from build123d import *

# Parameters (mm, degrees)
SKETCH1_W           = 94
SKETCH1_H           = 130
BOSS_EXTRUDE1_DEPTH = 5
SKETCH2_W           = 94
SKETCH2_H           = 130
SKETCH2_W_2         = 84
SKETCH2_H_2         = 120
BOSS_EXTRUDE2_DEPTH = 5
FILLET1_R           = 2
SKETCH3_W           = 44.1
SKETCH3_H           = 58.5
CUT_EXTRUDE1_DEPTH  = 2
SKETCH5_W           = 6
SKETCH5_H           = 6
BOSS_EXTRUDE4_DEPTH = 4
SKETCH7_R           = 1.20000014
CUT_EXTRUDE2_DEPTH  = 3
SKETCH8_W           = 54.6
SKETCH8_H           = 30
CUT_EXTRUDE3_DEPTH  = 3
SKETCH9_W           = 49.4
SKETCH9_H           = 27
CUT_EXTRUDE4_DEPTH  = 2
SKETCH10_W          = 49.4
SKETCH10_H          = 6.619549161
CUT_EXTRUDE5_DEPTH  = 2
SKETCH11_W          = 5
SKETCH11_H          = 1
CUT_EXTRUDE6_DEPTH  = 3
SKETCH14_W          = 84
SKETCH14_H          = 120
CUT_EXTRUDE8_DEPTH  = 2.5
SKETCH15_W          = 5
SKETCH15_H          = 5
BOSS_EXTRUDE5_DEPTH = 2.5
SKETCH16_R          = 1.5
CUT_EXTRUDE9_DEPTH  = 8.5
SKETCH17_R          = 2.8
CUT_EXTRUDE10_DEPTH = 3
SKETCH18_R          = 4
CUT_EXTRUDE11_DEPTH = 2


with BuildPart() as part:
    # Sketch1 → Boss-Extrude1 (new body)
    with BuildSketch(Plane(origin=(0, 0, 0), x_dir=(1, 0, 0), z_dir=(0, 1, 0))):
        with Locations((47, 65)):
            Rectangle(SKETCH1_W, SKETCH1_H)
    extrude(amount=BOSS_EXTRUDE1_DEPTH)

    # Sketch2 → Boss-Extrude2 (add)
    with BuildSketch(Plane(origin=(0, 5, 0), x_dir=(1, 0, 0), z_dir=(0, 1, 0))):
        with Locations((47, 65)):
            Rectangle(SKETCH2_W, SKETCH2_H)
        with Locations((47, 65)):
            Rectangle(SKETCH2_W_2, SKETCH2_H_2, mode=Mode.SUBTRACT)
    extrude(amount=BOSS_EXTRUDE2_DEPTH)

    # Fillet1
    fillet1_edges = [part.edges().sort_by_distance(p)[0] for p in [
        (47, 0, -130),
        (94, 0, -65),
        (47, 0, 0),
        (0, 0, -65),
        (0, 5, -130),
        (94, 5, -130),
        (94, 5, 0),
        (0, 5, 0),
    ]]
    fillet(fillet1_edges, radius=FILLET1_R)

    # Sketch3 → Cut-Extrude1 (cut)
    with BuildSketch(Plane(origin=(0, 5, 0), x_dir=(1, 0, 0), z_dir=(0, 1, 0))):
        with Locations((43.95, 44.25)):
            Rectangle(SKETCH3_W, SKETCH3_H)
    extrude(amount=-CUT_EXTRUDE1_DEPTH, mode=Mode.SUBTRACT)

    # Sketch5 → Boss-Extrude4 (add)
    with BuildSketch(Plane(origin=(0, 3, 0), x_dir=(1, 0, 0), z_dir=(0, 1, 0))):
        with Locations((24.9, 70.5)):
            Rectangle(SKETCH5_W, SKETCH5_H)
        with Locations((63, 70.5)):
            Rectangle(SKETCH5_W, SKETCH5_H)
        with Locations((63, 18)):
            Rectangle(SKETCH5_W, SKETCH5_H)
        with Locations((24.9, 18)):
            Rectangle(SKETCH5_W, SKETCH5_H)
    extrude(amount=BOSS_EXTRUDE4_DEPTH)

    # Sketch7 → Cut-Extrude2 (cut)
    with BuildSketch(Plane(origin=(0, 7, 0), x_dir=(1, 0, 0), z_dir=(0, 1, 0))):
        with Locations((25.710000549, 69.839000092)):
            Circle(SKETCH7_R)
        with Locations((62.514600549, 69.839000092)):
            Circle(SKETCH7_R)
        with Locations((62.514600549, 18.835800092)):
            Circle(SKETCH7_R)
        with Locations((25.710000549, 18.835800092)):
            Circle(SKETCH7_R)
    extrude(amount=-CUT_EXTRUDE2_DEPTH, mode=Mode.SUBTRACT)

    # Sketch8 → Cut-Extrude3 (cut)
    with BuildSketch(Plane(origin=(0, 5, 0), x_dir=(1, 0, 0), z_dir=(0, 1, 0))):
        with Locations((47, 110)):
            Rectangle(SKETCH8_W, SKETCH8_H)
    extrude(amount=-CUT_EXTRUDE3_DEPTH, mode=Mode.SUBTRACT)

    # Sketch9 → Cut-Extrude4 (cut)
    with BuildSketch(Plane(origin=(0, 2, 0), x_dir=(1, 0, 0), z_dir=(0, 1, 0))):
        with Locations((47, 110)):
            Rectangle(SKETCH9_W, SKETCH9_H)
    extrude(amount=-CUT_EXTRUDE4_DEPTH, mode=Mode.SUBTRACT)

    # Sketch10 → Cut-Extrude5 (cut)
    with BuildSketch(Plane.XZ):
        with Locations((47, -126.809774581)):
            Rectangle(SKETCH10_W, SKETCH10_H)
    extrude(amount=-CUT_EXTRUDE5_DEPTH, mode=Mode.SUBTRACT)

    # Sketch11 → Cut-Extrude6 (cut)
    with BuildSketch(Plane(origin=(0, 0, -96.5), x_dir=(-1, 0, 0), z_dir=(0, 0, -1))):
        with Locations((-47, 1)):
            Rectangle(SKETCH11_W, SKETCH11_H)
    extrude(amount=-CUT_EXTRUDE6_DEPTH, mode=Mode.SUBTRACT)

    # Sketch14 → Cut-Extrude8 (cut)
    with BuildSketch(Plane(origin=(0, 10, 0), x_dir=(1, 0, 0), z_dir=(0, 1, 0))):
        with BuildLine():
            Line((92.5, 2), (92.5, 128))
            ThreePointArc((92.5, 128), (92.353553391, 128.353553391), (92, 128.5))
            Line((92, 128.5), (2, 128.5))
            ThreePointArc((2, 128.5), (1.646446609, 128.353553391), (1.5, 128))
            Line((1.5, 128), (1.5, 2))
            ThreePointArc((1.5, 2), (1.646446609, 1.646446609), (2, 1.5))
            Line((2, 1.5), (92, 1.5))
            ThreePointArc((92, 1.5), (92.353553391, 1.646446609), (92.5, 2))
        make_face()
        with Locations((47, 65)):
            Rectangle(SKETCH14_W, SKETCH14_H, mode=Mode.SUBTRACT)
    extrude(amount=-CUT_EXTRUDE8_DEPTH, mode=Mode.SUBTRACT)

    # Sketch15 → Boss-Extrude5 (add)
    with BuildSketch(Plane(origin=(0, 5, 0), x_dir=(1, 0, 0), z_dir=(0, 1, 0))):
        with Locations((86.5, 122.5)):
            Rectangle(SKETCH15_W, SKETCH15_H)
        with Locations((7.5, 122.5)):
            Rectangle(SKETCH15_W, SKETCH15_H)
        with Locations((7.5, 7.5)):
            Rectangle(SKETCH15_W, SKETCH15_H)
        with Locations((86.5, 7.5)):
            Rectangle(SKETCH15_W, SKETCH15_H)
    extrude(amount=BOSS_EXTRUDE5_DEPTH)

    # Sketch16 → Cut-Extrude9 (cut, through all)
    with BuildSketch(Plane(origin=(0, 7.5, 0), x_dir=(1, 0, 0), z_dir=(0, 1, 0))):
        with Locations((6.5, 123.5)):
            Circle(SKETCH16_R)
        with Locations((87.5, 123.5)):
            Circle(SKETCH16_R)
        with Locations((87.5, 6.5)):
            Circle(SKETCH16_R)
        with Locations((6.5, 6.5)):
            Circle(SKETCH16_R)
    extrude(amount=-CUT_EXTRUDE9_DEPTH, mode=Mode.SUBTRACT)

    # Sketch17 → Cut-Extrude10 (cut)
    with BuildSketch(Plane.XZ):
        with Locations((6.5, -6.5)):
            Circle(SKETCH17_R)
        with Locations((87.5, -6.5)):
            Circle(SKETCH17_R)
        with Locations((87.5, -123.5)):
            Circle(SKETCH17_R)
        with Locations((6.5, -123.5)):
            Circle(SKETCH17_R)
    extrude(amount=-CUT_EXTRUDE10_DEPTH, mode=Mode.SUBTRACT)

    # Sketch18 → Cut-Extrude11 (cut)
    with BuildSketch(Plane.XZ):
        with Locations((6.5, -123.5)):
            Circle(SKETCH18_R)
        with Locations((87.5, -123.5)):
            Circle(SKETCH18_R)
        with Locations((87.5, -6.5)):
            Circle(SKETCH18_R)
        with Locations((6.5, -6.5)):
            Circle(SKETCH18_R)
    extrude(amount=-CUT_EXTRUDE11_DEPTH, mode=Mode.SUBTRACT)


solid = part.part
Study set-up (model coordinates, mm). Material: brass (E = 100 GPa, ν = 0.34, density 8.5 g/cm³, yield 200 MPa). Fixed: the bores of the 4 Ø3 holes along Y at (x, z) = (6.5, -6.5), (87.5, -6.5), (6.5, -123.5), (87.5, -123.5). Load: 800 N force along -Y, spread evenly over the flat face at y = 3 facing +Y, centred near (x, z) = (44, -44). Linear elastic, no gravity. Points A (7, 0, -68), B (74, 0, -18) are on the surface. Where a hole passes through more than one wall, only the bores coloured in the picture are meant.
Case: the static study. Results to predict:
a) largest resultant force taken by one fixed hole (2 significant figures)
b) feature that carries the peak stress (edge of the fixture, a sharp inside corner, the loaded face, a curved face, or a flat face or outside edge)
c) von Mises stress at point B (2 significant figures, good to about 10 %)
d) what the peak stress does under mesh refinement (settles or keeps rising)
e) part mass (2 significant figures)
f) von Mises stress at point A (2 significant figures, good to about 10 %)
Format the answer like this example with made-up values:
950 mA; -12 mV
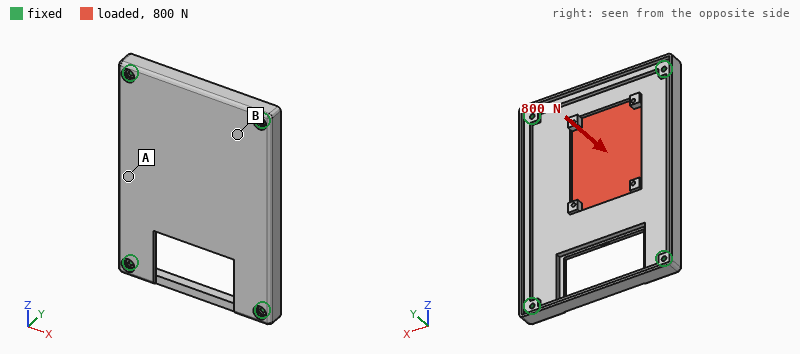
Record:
800 N; edge of the fixture; 6.9 MPa; keeps rising; 460 g; 17 MPa
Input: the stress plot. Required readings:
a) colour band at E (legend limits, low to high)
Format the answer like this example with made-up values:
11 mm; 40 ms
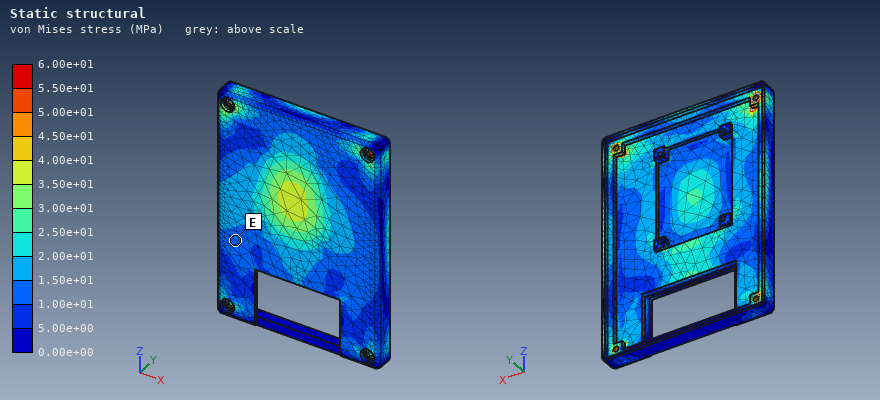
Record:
1.00e+01 to 1.50e+01 MPa
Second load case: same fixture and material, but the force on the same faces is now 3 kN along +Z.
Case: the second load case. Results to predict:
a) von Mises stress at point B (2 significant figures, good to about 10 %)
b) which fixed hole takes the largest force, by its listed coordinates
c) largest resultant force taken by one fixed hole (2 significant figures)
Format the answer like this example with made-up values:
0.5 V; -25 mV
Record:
5.5 MPa; (6.5, -6.5); 970 N
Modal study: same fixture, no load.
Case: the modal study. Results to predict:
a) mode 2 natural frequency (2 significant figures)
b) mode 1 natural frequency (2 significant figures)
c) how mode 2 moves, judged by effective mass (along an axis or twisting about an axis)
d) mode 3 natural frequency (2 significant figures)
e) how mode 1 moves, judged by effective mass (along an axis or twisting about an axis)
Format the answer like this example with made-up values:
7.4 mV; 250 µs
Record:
1500 Hz; 1000 Hz; twisting about Z; 2300 Hz; along Y
